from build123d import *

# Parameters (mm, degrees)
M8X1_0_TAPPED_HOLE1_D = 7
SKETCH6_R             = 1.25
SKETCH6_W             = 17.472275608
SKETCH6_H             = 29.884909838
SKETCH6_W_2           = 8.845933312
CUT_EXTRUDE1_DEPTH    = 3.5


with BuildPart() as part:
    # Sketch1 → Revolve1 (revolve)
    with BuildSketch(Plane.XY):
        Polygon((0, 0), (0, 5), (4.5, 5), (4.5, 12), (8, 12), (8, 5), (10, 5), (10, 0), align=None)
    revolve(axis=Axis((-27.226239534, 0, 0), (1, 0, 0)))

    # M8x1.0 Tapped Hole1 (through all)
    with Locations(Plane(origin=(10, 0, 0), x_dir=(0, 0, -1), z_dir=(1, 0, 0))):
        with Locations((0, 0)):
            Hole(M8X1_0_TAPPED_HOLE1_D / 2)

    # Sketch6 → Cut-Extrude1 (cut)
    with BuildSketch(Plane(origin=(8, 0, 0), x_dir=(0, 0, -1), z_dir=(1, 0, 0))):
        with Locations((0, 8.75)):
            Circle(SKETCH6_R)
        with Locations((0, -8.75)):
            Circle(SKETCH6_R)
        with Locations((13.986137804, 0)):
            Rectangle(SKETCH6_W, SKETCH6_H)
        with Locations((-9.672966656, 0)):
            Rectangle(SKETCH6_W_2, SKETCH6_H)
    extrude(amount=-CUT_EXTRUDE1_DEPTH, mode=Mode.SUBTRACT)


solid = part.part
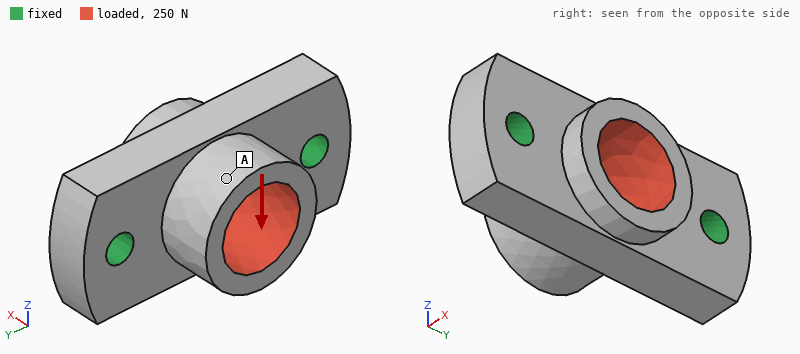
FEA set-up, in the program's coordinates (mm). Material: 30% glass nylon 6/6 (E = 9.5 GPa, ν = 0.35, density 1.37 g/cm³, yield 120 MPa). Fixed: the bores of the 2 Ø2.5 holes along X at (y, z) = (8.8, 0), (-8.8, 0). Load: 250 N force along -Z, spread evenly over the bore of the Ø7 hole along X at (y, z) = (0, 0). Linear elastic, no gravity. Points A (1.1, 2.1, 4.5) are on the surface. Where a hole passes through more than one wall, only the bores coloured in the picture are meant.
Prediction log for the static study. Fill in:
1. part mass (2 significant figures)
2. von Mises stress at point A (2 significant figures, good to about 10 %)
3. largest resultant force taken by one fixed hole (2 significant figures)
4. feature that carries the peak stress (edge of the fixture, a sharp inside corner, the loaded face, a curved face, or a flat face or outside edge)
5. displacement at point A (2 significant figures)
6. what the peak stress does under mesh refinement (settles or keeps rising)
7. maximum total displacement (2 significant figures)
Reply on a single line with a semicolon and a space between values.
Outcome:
1.3 g; 2.9 MPa; 130 N; edge of the fixture; 23 µm; keeps rising; 27 µm
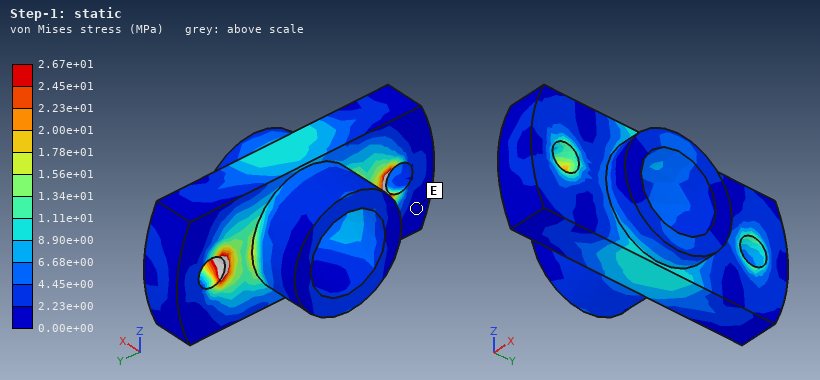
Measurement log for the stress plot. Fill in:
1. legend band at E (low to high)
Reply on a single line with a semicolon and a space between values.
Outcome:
0.00e+00 to 2.23e+00 MPa
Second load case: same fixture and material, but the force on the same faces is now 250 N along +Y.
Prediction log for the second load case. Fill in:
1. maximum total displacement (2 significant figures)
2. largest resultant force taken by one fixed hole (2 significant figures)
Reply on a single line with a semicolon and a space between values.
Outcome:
10 µm; 130 N
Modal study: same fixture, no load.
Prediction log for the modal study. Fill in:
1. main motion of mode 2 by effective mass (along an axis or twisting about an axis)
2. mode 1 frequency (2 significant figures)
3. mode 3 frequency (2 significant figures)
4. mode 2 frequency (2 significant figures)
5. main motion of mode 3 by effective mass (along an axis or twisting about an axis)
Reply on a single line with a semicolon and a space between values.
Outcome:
along X; 18 kHz; 32 kHz; 23 kHz; along Z
